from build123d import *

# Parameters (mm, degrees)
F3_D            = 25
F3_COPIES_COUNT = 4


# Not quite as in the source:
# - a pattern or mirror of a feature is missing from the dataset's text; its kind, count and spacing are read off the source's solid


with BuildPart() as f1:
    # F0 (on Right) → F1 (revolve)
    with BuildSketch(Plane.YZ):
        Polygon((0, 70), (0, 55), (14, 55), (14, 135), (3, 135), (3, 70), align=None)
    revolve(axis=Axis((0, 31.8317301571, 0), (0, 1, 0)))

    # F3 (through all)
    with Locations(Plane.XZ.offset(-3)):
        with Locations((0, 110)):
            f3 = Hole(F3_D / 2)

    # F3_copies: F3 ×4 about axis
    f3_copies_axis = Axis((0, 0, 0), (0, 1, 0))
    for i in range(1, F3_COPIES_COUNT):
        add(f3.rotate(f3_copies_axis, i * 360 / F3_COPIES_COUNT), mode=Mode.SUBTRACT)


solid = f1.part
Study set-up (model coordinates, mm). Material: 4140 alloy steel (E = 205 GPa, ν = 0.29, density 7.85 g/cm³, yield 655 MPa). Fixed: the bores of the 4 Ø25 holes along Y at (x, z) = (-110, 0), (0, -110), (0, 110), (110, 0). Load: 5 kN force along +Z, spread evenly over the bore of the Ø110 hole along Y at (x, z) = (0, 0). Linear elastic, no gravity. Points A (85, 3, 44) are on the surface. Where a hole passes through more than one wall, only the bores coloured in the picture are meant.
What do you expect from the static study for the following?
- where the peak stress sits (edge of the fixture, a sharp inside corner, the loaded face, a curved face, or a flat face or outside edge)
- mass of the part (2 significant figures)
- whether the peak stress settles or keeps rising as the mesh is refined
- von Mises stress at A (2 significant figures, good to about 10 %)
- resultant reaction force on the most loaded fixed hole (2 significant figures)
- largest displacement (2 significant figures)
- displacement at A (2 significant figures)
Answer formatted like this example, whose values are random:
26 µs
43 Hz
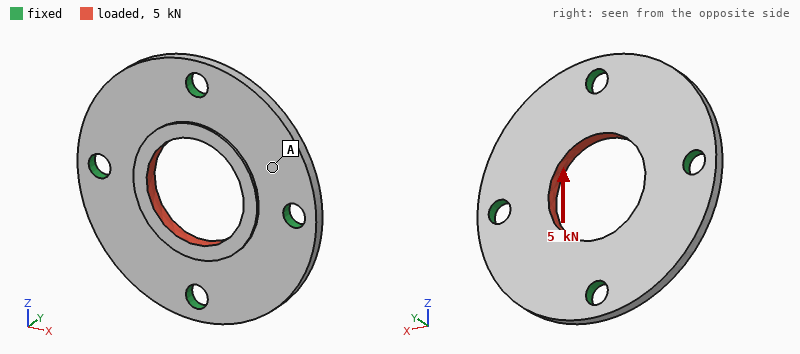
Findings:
edge of the fixture
4.1 kg
keeps rising
0.89 MPa
1.4 kN
0.81 µm
0.42 µm
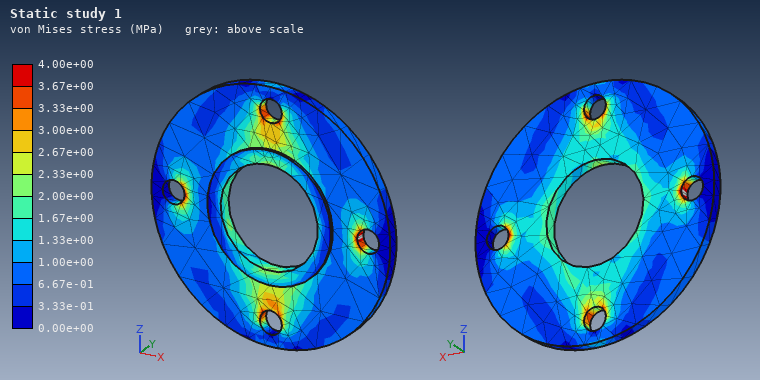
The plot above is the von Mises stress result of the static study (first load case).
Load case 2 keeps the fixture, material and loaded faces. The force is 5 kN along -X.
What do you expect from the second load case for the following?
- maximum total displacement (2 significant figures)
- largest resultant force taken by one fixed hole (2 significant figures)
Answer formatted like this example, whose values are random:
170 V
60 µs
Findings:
0.81 µm
1.4 kN
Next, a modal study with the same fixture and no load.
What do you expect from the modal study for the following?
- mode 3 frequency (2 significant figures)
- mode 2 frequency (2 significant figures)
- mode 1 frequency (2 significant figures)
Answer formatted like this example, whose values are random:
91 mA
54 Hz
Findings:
2300 Hz
2300 Hz
2200 Hz
